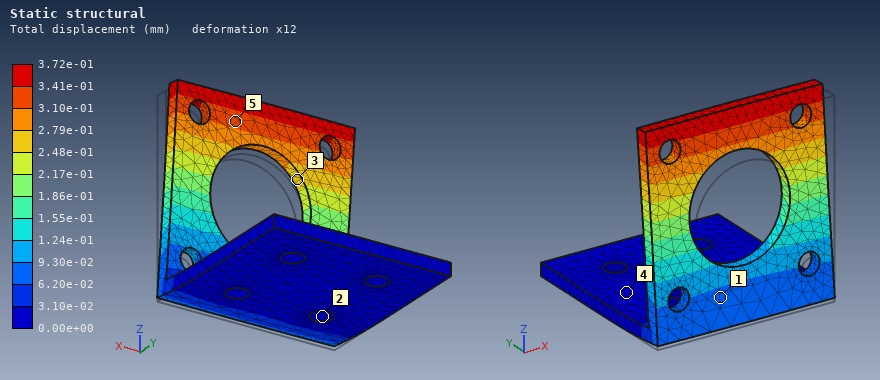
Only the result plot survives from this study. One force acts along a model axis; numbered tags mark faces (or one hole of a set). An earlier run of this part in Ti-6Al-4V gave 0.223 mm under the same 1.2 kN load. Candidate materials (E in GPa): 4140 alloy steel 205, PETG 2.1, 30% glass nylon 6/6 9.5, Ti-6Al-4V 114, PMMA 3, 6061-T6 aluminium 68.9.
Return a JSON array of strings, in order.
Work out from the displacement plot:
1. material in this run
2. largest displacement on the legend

["6061-T6 aluminium", "3.72e-01 mm"]
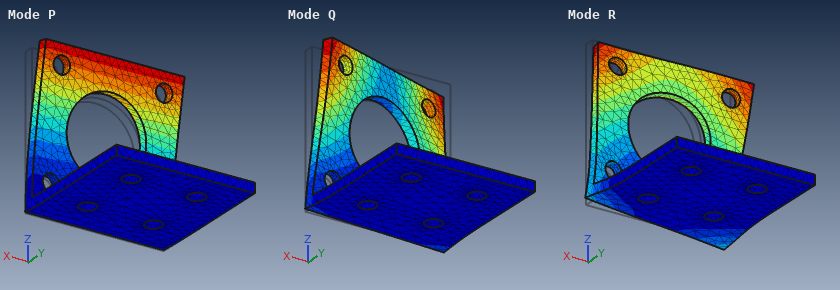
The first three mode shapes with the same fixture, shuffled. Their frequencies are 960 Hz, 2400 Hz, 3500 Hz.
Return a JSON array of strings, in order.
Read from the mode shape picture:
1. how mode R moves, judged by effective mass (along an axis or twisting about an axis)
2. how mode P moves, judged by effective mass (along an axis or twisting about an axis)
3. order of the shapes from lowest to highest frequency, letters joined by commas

["along X", "along Y", "P, Q, R"]
